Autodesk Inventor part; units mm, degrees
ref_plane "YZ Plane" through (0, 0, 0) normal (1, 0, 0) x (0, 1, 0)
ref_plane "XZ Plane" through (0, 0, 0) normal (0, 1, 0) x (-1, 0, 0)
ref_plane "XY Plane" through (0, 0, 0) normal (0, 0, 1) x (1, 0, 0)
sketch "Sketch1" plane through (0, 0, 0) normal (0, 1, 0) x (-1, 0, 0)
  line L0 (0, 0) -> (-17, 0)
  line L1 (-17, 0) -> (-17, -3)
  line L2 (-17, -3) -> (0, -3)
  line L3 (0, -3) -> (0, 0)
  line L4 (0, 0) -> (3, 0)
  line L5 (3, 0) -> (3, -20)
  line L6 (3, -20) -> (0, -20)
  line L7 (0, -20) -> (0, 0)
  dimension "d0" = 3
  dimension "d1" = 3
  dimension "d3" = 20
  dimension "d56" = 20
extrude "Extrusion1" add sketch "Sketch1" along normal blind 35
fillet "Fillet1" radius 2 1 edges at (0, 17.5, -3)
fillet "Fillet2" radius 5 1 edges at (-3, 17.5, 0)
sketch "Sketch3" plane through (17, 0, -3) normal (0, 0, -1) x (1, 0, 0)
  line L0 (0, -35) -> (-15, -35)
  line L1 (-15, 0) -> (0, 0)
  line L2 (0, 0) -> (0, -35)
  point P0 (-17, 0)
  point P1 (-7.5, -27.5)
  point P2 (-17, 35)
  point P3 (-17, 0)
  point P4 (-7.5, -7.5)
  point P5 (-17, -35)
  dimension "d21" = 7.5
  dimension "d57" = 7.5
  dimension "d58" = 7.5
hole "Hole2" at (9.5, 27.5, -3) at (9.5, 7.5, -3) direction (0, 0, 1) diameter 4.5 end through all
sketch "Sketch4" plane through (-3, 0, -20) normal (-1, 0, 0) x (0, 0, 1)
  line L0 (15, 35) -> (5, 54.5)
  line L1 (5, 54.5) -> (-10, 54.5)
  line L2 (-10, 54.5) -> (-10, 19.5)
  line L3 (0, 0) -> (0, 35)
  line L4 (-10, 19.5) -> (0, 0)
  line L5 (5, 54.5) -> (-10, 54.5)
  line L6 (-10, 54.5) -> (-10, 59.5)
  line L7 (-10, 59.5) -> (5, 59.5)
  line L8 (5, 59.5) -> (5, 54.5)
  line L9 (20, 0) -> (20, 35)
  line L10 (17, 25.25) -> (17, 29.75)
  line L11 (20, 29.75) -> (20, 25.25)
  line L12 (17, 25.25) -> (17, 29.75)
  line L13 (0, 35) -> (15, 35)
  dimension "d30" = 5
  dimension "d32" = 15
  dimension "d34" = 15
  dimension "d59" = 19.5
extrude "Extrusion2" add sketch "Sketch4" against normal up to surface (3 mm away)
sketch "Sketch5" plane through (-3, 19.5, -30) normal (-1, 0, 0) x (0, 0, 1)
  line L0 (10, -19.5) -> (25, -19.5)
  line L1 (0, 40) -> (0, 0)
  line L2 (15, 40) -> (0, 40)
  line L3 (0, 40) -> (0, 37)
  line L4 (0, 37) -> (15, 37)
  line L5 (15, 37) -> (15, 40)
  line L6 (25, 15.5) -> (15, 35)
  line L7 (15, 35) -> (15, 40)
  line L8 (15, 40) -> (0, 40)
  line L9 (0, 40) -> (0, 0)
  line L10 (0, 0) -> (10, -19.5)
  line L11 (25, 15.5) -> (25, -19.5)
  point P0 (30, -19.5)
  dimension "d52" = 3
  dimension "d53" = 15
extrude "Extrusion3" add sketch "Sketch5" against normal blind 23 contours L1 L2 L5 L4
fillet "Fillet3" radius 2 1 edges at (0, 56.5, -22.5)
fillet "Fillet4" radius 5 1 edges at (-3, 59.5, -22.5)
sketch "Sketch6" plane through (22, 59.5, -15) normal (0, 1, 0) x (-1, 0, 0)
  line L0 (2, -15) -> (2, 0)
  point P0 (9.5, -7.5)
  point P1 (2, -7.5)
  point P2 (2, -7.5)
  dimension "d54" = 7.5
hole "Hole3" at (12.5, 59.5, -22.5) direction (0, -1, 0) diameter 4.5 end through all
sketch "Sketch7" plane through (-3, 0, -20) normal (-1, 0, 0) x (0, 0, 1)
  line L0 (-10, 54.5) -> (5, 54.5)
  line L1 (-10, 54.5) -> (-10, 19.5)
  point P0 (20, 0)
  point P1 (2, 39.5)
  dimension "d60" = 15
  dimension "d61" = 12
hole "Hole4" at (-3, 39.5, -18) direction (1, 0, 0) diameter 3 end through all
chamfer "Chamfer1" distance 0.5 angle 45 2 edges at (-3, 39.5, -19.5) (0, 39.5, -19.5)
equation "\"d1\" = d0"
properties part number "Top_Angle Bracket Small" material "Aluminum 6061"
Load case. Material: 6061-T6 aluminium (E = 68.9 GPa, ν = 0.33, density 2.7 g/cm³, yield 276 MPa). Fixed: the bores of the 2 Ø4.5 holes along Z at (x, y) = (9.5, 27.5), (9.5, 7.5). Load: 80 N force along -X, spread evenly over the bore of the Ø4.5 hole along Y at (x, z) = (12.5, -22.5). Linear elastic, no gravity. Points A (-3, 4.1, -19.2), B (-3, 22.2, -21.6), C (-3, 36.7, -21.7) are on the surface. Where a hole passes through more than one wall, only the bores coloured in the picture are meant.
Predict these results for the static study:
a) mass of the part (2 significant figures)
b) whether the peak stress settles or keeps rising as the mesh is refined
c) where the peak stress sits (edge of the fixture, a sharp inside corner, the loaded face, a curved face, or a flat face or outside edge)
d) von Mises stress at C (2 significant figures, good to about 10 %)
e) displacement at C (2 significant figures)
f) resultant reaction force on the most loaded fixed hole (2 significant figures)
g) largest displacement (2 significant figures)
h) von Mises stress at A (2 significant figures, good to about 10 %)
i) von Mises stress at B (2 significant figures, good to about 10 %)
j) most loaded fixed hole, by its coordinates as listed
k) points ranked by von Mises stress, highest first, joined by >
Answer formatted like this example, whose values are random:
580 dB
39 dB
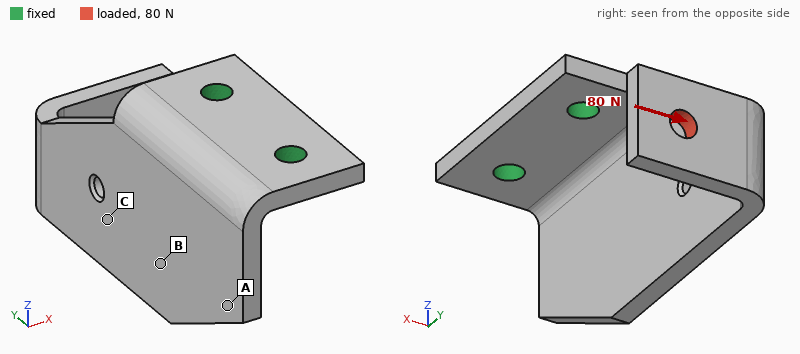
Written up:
18 g
keeps rising
a sharp inside corner
52 MPa
0.20 mm
180 N
0.70 mm
14 MPa
35 MPa
(9.5, 27.5)
C > B > A
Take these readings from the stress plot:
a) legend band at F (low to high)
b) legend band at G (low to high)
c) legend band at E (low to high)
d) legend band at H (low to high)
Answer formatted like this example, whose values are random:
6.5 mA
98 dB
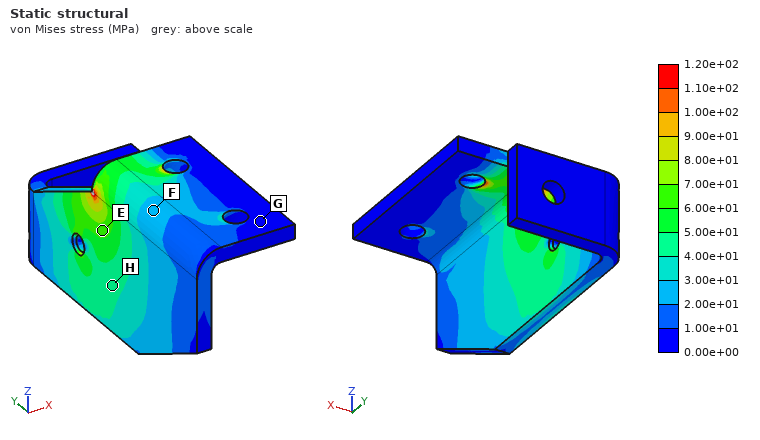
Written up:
2.00e+01 to 3.00e+01 MPa
0.00e+00 to 1.00e+01 MPa
6.00e+01 to 7.00e+01 MPa
4.00e+01 to 5.00e+01 MPa
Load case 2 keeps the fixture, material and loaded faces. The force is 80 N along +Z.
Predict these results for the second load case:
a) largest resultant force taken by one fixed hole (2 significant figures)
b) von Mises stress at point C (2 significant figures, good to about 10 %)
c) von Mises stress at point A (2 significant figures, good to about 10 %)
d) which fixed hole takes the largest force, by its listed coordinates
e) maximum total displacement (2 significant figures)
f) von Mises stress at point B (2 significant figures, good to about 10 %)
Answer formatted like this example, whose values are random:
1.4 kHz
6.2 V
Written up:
180 N
27 MPa
7.7 MPa
(9.5, 27.5)
0.33 mm
17 MPa
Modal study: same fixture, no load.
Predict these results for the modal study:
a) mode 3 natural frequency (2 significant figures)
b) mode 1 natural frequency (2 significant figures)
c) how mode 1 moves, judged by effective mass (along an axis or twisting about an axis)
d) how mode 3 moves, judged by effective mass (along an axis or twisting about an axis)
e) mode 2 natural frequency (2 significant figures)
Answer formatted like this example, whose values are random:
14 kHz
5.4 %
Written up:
2500 Hz
950 Hz
along X
along Z
1900 Hz
